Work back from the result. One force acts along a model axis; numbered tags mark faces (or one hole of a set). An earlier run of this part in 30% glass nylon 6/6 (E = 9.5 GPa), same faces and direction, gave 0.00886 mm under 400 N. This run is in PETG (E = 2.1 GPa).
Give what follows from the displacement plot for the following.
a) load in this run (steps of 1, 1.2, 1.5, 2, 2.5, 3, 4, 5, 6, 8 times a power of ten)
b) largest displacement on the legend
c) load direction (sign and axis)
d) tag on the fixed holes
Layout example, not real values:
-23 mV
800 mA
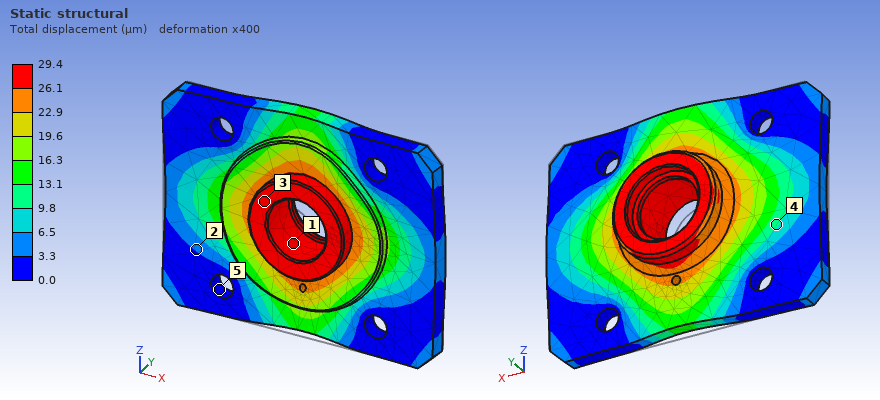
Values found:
300 N
29.4 µm
+Y
5
